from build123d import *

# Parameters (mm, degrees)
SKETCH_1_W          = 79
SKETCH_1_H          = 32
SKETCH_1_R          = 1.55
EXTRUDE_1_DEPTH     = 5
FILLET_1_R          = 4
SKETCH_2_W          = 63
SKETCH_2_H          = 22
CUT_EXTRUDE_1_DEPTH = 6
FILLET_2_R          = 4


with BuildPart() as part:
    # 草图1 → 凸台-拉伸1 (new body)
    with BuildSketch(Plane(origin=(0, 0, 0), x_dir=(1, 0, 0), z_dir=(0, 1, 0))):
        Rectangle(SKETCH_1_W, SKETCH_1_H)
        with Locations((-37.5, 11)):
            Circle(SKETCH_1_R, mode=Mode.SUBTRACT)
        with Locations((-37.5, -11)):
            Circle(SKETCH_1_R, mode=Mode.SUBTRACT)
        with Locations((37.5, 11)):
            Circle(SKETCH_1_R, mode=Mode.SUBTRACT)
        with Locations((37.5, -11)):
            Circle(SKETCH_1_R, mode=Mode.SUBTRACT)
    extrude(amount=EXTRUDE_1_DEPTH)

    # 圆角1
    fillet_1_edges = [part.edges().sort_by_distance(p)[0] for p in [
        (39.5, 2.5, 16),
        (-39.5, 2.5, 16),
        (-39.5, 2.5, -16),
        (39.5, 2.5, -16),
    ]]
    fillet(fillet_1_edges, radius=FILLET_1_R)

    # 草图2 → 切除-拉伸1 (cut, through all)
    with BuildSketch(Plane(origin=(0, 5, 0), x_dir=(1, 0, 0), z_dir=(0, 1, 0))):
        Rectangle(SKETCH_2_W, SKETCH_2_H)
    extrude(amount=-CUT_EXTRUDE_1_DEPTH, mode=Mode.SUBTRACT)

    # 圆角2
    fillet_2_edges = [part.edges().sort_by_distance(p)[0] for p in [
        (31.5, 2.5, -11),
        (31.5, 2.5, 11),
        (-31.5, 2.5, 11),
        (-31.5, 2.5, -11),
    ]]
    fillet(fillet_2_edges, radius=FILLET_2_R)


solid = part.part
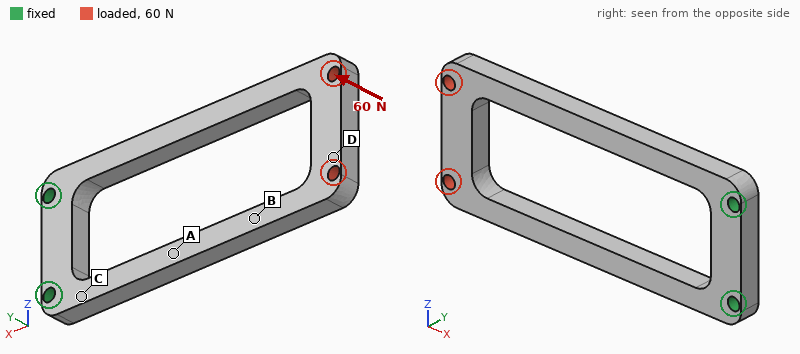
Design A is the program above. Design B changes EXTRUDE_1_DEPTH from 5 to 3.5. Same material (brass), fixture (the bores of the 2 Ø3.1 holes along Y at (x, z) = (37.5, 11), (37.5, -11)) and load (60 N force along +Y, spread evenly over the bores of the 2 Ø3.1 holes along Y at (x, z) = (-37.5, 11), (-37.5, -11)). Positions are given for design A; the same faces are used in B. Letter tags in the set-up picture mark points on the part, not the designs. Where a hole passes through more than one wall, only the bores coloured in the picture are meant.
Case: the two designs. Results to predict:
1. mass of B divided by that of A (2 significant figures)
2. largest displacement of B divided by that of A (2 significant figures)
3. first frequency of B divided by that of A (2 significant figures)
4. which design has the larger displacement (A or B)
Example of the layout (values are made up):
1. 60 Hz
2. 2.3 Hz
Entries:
1. 0.70
2. 2.9
3. 0.71
4. B
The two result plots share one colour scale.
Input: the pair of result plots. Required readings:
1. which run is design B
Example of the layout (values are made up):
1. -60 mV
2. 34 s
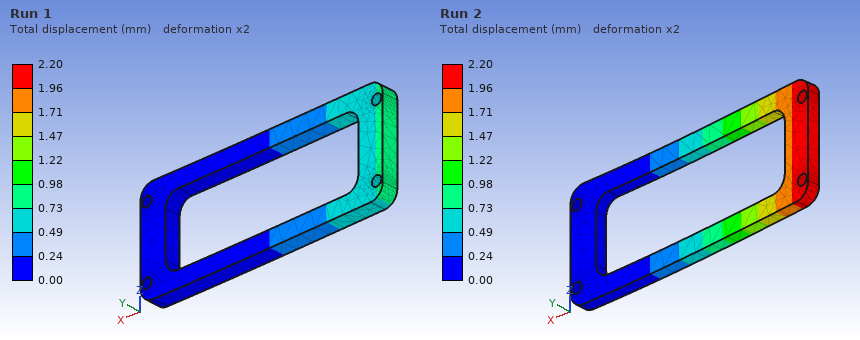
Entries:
1. Run 2
